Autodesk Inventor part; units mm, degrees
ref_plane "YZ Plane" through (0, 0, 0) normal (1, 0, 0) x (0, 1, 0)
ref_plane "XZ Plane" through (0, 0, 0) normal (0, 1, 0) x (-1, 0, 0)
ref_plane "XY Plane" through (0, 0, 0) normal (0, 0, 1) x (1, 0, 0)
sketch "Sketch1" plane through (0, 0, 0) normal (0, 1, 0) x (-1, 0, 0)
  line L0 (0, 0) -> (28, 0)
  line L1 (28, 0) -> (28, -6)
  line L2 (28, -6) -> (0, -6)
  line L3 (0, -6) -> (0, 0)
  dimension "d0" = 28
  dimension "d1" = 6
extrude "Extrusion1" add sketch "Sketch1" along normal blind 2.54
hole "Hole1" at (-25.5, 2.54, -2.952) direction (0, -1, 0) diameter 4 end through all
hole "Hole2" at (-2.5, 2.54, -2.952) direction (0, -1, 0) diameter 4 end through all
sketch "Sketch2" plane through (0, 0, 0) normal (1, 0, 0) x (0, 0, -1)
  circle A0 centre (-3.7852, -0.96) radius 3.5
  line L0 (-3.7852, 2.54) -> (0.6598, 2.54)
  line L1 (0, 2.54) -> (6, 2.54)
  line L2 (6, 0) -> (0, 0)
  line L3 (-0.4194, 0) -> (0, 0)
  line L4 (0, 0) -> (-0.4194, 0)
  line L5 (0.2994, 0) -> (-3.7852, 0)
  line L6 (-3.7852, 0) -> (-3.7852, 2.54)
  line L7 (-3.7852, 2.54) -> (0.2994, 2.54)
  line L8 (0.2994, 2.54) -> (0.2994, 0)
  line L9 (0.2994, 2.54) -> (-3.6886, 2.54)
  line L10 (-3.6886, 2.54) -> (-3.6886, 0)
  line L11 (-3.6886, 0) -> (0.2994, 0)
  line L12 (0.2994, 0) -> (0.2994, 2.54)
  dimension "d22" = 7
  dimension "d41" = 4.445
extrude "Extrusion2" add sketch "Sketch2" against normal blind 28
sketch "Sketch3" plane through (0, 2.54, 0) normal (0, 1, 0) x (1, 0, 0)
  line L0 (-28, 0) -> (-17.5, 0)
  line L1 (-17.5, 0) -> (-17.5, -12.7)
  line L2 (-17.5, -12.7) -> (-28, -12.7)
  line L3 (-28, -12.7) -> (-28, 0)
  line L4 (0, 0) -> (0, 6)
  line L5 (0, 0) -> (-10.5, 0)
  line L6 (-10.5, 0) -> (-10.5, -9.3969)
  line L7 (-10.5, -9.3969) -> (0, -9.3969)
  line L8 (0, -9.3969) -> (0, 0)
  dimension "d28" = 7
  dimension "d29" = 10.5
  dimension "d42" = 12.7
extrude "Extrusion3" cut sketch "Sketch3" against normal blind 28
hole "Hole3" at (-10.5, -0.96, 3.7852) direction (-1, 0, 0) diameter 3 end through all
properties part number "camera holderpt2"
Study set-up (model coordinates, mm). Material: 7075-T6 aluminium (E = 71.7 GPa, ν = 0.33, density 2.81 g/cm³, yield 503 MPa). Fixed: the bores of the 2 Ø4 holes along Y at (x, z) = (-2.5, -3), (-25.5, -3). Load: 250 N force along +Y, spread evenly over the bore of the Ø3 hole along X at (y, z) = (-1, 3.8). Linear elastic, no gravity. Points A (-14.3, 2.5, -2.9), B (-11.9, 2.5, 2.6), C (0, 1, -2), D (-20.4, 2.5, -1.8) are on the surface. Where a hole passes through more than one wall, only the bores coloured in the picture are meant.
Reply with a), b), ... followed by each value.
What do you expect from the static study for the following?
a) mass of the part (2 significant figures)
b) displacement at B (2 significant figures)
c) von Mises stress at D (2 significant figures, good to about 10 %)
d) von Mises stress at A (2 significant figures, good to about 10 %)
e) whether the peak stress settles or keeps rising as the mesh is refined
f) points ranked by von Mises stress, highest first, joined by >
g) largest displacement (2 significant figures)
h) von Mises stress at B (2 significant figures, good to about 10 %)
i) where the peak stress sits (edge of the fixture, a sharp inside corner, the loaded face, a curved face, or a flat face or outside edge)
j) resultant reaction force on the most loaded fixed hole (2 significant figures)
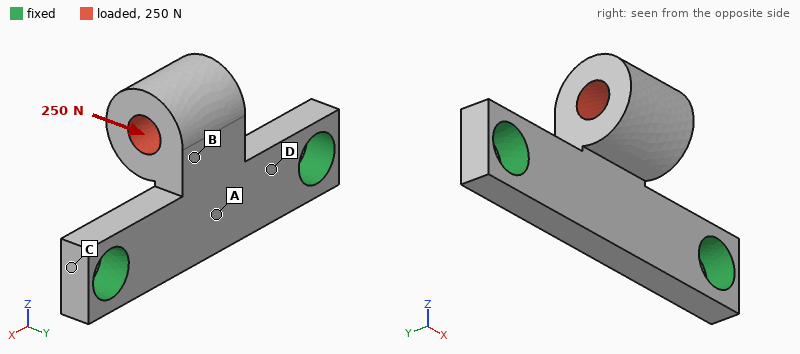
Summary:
a) 1.7 g
b) 0.080 mm
c) 140 MPa
d) 75 MPa
e) keeps rising
f) D > A > B > C
g) 0.15 mm
h) 41 MPa
i) a sharp inside corner
j) 130 N
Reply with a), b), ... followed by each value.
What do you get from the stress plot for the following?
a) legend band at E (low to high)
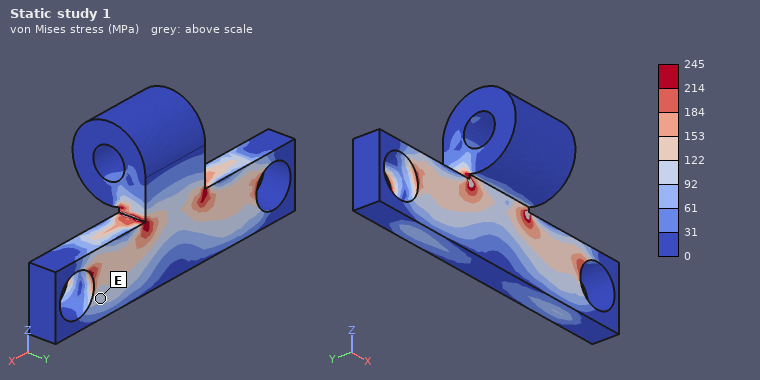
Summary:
a) 92 to 122 MPa
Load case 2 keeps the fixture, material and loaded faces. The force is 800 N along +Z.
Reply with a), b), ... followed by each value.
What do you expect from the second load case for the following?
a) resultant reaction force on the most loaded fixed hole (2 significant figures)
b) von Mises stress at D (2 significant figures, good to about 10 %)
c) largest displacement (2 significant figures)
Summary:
a) 410 N
b) 81 MPa
c) 0.18 mm
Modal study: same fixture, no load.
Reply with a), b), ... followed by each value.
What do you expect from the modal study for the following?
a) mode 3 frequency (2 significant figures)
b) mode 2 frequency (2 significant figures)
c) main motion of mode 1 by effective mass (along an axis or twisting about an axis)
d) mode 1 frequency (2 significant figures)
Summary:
a) 26 kHz
b) 26 kHz
c) along Y
d) 8900 Hz
